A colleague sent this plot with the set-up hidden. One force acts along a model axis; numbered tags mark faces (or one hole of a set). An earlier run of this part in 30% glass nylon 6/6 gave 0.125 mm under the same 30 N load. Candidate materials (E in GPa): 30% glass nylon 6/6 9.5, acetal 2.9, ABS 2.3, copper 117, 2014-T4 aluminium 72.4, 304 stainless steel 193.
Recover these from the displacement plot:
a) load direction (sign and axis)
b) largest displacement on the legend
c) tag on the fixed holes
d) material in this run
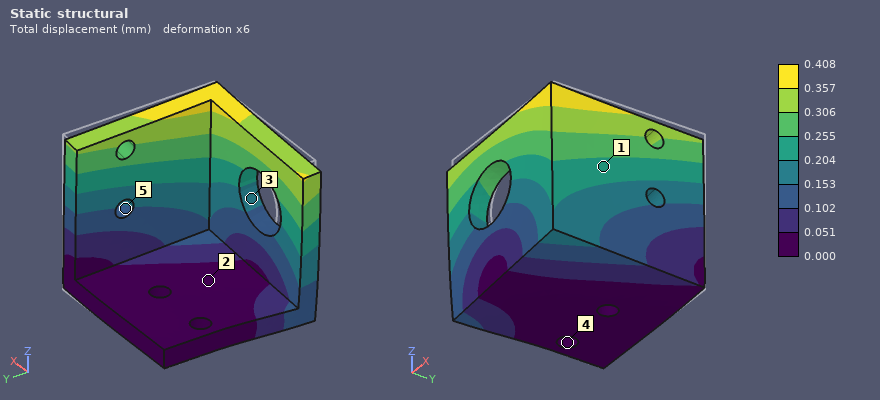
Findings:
-X
0.408 mm
4
acetal
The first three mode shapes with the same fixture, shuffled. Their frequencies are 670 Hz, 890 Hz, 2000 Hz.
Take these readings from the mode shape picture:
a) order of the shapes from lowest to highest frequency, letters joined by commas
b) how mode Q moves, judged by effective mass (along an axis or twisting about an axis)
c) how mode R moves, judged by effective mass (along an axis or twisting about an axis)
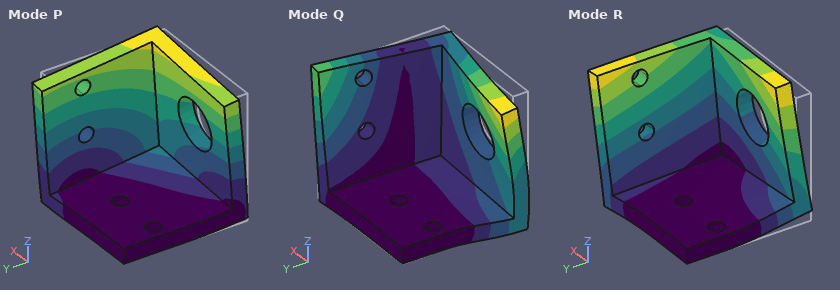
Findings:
P, R, Q
along Z
along X
